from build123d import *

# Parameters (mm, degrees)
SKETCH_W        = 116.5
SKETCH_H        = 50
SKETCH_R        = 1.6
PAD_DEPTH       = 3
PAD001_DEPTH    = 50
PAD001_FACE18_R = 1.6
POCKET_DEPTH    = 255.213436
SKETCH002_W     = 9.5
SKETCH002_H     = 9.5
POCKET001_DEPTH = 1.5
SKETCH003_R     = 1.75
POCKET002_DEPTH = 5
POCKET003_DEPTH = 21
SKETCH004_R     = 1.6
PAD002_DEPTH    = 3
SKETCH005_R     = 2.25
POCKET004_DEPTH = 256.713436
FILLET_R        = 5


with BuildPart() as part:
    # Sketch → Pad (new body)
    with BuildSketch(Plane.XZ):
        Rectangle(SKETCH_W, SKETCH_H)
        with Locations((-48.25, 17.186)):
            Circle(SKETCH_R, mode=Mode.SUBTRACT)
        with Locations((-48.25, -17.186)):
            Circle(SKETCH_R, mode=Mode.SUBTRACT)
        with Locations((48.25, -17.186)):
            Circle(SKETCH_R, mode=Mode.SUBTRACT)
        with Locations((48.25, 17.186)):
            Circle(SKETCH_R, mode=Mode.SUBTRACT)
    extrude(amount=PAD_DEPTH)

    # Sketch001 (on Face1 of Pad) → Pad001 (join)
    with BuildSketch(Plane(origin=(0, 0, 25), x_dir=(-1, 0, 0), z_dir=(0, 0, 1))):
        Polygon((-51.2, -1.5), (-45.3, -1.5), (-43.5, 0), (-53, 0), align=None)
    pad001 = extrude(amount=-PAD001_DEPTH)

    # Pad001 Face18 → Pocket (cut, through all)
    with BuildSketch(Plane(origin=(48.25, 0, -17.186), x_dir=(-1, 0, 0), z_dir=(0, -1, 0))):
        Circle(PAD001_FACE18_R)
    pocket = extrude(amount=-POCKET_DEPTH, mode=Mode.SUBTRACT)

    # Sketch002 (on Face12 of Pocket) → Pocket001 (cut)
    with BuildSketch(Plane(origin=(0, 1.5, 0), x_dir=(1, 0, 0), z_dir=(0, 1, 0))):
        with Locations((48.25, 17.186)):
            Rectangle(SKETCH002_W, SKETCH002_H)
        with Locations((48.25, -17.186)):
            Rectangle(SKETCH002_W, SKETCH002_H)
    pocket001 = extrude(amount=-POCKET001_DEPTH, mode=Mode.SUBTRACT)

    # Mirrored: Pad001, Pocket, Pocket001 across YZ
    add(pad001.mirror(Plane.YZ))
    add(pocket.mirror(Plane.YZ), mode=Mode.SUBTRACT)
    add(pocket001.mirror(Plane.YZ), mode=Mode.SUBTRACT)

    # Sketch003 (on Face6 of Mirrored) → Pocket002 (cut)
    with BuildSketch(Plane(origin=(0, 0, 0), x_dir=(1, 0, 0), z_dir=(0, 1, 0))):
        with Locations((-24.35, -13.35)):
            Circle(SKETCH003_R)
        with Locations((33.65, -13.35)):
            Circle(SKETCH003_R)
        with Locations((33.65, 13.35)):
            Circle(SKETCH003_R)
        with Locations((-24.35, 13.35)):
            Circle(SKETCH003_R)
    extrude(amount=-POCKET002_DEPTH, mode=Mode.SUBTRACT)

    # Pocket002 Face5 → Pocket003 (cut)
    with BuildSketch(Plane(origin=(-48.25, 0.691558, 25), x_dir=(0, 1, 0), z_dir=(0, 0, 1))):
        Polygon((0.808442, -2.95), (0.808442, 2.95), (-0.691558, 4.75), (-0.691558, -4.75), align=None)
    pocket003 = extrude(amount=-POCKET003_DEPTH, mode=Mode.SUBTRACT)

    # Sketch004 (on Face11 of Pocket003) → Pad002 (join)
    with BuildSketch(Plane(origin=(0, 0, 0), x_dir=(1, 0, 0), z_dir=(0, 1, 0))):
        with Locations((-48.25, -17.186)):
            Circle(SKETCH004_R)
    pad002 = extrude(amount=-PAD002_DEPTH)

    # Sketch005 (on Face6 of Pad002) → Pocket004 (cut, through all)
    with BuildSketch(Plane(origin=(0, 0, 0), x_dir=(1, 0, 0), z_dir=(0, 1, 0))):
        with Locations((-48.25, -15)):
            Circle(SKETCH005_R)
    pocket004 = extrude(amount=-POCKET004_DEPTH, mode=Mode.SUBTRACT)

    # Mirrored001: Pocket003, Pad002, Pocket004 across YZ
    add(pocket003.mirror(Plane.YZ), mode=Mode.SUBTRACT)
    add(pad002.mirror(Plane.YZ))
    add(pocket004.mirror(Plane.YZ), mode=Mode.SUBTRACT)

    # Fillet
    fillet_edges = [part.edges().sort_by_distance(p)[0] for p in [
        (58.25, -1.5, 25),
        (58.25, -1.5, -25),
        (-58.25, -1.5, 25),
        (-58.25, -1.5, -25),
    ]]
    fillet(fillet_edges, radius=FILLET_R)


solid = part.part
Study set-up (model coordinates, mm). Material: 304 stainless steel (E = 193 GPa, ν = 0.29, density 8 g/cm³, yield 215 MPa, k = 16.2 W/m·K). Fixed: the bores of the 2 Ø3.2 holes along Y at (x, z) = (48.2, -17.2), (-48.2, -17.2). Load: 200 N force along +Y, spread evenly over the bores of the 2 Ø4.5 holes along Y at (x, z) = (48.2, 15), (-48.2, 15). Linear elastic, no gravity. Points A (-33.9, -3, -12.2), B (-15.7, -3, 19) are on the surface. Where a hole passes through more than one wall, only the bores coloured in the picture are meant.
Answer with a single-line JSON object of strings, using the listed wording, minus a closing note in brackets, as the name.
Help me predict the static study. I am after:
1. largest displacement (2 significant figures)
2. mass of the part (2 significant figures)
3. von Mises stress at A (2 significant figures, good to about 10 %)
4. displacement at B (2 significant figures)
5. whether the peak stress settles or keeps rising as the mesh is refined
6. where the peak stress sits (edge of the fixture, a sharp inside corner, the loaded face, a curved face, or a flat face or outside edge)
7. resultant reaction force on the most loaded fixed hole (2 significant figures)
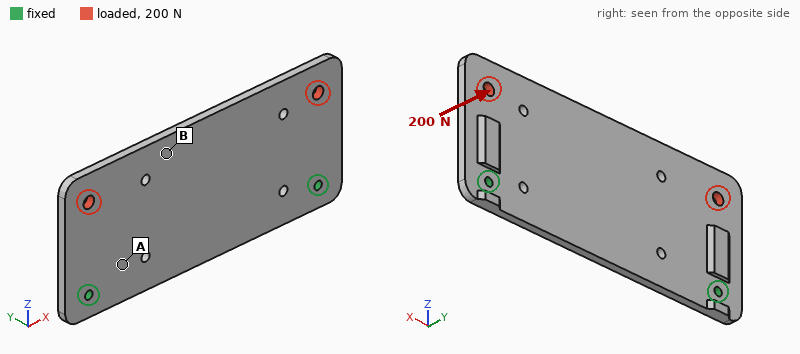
{"largest displacement": "0.12 mm", "mass of the part": "140 g", "von Mises stress at A": "25 MPa", "displacement at B": "0.088 mm", "whether the peak stress settles or keeps rising as the mesh is refined": "keeps rising", "where the peak stress sits": "edge of the fixture", "resultant reaction force on the most loaded fixed hole": "100 N"}
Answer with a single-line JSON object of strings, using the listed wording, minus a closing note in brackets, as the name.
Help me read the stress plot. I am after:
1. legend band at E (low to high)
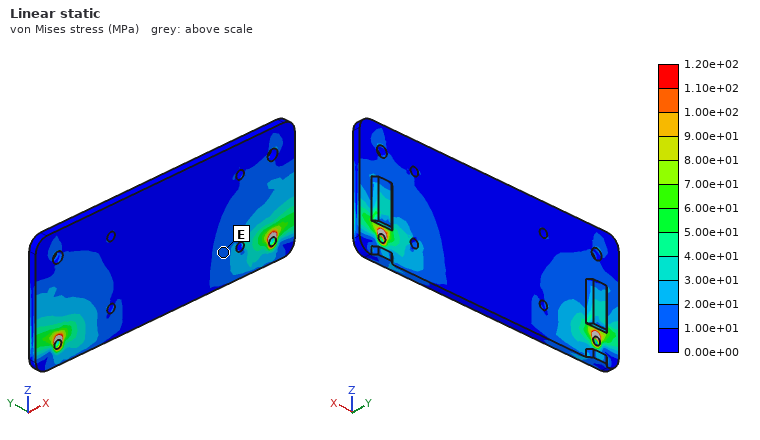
{"legend band at E": "1.00e+01 to 2.00e+01 MPa"}
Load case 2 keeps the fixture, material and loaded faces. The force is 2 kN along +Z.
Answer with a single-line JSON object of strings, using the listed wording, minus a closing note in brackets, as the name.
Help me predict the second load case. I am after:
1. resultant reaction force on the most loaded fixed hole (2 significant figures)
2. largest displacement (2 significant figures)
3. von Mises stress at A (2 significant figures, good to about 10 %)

{"resultant reaction force on the most loaded fixed hole": "1.0 kN", "largest displacement": "6.1 µm", "von Mises stress at A": "4.9 MPa"}
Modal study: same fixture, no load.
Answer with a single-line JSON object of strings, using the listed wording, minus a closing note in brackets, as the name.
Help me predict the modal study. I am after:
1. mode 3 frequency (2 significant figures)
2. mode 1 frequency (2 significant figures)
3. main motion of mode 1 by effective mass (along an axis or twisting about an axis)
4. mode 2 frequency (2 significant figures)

{"mode 3 frequency": "1800 Hz", "mode 1 frequency": "850 Hz", "main motion of mode 1 by effective mass": "along Y", "mode 2 frequency": "1700 Hz"}
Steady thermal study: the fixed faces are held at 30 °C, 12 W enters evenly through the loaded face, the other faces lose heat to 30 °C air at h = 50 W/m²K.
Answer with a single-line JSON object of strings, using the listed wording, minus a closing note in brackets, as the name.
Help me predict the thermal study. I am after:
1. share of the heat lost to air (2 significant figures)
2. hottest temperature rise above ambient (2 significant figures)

{"share of the heat lost to air": "82 %", "hottest temperature rise above ambient": "75 K"}
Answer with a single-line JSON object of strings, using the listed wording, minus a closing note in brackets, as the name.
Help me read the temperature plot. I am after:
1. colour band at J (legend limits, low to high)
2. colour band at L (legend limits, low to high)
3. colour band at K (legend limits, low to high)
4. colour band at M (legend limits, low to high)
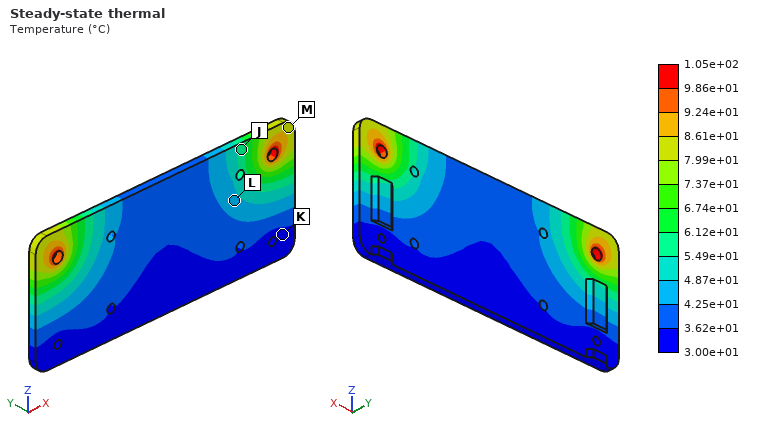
{"colour band at J": "5.49e+01 to 6.12e+01 °C", "colour band at L": "4.25e+01 to 4.87e+01 °C", "colour band at K": "3.00e+01 to 3.62e+01 °C", "colour band at M": "7.99e+01 to 8.61e+01 °C"}
